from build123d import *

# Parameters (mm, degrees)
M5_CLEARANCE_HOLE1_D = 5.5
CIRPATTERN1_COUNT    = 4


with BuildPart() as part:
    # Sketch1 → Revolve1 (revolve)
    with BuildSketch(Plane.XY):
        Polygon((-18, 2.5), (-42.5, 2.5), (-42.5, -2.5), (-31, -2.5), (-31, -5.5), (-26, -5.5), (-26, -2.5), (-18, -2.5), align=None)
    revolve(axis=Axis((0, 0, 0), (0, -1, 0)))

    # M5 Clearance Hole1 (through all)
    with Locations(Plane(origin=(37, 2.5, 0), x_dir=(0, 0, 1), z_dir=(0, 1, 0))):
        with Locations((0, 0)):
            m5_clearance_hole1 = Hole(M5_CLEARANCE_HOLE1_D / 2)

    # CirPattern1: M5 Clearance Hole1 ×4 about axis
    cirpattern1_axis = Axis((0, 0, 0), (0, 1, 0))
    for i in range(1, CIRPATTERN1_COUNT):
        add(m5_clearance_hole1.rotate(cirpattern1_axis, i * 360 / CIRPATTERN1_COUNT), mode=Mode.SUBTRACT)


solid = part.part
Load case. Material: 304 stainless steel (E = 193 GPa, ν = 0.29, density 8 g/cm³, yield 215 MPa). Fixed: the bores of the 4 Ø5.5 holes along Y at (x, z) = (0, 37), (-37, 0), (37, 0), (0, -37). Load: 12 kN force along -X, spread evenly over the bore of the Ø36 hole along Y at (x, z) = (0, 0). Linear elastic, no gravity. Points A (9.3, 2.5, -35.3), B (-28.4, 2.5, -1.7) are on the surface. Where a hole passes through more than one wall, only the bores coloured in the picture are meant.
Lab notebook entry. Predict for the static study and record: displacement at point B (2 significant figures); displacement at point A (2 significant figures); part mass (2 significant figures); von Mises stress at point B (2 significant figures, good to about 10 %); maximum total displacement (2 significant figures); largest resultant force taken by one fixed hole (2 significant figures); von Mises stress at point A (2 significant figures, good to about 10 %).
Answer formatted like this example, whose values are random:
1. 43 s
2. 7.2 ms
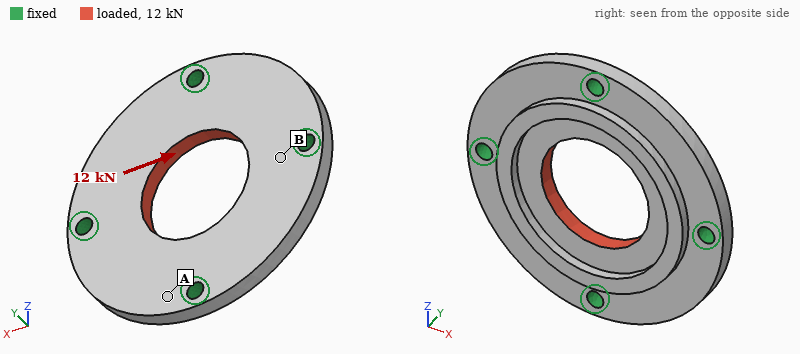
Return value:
1. 1.6 µm
2. 1.5 µm
3. 200 g
4. 46 MPa
5. 5.4 µm
6. 3.3 kN
7. 23 MPa
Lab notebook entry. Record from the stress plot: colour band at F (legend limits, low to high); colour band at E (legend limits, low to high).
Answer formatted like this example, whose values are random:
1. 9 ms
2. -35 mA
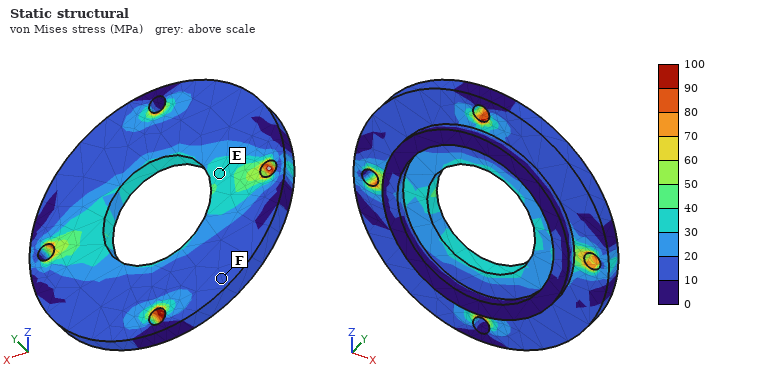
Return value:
1. 10 to 20 MPa
2. 30 to 40 MPa
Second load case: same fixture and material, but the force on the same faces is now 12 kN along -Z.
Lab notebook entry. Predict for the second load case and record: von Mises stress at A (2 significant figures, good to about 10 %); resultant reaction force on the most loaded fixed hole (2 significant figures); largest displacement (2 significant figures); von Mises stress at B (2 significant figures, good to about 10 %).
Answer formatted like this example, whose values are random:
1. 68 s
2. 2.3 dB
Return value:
1. 15 MPa
2. 3.3 kN
3. 5.4 µm
4. 13 MPa
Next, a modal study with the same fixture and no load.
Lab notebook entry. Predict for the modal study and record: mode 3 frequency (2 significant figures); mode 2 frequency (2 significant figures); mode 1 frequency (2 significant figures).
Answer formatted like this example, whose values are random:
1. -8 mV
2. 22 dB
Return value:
1. 8700 Hz
2. 8700 Hz
3. 7900 Hz
